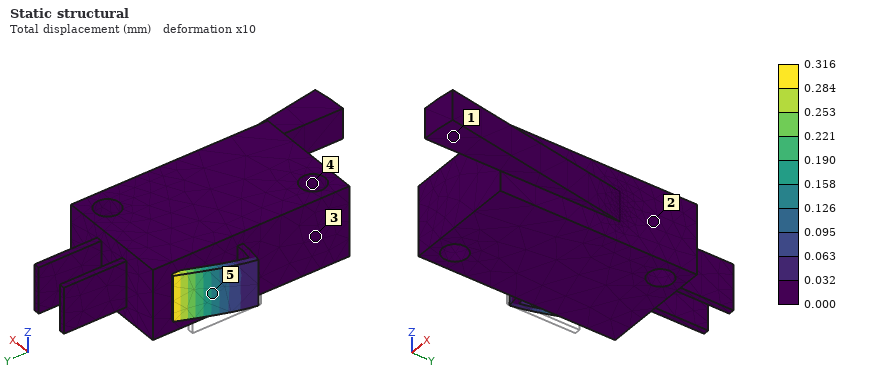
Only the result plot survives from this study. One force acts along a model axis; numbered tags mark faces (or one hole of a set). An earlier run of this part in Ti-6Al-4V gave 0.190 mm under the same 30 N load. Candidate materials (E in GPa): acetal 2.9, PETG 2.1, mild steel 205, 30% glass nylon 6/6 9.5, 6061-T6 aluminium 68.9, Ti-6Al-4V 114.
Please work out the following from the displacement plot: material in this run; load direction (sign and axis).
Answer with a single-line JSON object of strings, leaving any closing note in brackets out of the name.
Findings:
{"material in this run": "6061-T6 aluminium", "load direction": "+X"}
